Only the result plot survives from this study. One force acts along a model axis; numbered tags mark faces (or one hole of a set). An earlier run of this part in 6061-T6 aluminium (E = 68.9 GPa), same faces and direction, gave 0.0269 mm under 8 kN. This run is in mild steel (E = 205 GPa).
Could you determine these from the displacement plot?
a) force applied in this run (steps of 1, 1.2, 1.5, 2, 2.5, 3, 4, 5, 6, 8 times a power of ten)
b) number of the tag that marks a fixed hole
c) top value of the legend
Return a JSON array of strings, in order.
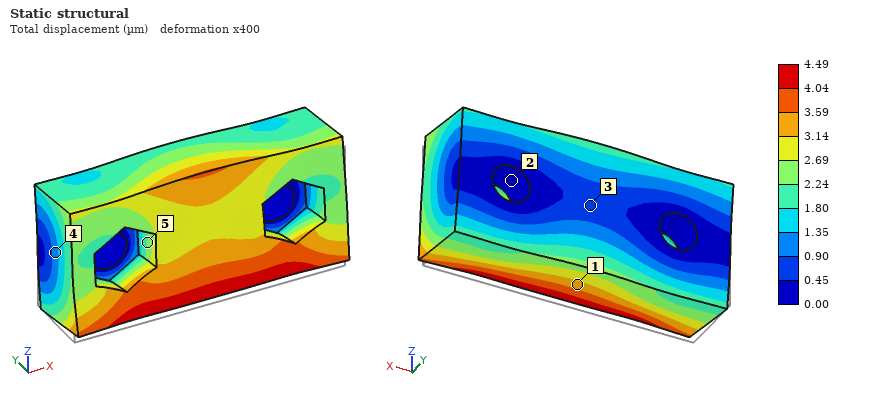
["4 kN", "2", "4.49 µm"]
